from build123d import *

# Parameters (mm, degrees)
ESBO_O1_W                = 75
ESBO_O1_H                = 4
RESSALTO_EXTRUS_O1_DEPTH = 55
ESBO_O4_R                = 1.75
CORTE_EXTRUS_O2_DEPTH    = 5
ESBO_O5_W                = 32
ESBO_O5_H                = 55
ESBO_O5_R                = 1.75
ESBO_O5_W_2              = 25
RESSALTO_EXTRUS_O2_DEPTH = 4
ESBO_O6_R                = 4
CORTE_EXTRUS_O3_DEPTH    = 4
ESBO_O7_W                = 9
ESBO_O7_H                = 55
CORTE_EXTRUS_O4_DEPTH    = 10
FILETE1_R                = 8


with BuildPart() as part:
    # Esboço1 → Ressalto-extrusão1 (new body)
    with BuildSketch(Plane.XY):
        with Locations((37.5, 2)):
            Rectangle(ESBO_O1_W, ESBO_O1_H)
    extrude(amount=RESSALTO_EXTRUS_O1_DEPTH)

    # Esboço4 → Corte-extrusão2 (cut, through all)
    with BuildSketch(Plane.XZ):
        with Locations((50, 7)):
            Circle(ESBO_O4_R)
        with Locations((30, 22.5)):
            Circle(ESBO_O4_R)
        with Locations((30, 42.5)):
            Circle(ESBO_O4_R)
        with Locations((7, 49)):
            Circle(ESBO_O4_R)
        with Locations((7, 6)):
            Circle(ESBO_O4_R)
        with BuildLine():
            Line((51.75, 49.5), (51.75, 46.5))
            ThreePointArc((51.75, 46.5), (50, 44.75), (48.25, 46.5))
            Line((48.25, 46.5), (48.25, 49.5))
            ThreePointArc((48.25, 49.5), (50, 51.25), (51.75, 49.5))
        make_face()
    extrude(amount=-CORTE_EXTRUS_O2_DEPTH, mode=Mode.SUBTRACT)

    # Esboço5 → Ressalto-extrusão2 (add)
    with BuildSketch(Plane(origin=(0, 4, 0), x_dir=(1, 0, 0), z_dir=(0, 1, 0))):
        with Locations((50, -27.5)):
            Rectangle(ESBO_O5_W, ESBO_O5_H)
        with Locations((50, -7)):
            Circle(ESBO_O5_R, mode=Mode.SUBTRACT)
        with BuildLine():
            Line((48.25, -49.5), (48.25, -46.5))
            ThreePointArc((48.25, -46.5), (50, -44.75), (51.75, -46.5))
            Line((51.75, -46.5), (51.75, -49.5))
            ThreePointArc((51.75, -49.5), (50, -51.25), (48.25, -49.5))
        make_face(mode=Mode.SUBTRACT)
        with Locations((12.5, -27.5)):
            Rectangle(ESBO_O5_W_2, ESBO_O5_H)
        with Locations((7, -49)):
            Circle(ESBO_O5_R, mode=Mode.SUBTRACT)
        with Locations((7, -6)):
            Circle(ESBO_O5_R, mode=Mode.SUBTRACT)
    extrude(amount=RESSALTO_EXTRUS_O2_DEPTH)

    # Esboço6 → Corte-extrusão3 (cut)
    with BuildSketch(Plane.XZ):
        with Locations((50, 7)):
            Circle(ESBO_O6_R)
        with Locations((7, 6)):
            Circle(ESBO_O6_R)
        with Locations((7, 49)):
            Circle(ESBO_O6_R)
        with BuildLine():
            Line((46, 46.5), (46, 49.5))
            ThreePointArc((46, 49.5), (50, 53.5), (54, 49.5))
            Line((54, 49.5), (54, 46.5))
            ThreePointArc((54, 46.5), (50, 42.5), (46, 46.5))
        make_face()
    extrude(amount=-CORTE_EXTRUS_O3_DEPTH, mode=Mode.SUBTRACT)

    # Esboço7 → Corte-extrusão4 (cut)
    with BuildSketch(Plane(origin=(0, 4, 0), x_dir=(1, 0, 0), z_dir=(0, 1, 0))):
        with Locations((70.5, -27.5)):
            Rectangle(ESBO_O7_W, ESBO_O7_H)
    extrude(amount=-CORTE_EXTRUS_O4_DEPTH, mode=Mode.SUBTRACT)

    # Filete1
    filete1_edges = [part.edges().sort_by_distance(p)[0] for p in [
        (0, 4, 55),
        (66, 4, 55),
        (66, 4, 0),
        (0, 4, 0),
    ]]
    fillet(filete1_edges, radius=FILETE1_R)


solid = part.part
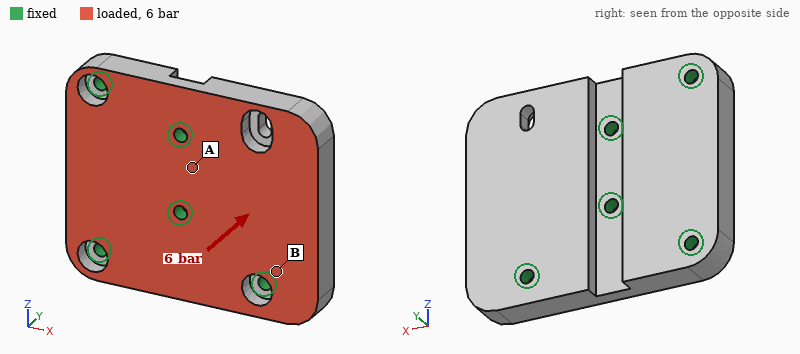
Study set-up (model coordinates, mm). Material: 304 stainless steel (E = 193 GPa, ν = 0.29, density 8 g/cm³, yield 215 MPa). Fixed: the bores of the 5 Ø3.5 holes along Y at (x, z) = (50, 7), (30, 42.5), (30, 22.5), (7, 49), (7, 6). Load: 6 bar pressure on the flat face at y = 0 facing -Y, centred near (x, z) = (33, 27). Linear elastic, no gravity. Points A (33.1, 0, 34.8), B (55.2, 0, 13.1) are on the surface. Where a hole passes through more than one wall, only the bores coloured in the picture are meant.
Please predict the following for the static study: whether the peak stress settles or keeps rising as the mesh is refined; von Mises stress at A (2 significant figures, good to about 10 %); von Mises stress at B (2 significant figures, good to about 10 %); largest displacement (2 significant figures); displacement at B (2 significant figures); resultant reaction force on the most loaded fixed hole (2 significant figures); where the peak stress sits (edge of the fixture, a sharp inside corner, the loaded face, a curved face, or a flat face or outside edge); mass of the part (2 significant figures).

keeps rising
24 MPa
9.1 MPa
24 µm
4.7 µm
650 N
edge of the fixture
200 g
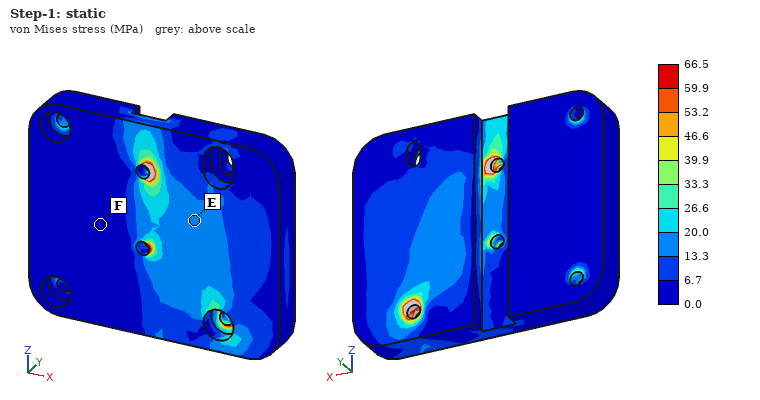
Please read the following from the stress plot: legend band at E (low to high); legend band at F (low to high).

13.3 to 20.0 MPa
0.0 to 6.7 MPa
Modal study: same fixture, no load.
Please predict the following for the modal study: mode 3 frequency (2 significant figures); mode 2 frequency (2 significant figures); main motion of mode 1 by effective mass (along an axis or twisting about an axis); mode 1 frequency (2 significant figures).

15 kHz
12 kHz
along Y
4100 Hz
